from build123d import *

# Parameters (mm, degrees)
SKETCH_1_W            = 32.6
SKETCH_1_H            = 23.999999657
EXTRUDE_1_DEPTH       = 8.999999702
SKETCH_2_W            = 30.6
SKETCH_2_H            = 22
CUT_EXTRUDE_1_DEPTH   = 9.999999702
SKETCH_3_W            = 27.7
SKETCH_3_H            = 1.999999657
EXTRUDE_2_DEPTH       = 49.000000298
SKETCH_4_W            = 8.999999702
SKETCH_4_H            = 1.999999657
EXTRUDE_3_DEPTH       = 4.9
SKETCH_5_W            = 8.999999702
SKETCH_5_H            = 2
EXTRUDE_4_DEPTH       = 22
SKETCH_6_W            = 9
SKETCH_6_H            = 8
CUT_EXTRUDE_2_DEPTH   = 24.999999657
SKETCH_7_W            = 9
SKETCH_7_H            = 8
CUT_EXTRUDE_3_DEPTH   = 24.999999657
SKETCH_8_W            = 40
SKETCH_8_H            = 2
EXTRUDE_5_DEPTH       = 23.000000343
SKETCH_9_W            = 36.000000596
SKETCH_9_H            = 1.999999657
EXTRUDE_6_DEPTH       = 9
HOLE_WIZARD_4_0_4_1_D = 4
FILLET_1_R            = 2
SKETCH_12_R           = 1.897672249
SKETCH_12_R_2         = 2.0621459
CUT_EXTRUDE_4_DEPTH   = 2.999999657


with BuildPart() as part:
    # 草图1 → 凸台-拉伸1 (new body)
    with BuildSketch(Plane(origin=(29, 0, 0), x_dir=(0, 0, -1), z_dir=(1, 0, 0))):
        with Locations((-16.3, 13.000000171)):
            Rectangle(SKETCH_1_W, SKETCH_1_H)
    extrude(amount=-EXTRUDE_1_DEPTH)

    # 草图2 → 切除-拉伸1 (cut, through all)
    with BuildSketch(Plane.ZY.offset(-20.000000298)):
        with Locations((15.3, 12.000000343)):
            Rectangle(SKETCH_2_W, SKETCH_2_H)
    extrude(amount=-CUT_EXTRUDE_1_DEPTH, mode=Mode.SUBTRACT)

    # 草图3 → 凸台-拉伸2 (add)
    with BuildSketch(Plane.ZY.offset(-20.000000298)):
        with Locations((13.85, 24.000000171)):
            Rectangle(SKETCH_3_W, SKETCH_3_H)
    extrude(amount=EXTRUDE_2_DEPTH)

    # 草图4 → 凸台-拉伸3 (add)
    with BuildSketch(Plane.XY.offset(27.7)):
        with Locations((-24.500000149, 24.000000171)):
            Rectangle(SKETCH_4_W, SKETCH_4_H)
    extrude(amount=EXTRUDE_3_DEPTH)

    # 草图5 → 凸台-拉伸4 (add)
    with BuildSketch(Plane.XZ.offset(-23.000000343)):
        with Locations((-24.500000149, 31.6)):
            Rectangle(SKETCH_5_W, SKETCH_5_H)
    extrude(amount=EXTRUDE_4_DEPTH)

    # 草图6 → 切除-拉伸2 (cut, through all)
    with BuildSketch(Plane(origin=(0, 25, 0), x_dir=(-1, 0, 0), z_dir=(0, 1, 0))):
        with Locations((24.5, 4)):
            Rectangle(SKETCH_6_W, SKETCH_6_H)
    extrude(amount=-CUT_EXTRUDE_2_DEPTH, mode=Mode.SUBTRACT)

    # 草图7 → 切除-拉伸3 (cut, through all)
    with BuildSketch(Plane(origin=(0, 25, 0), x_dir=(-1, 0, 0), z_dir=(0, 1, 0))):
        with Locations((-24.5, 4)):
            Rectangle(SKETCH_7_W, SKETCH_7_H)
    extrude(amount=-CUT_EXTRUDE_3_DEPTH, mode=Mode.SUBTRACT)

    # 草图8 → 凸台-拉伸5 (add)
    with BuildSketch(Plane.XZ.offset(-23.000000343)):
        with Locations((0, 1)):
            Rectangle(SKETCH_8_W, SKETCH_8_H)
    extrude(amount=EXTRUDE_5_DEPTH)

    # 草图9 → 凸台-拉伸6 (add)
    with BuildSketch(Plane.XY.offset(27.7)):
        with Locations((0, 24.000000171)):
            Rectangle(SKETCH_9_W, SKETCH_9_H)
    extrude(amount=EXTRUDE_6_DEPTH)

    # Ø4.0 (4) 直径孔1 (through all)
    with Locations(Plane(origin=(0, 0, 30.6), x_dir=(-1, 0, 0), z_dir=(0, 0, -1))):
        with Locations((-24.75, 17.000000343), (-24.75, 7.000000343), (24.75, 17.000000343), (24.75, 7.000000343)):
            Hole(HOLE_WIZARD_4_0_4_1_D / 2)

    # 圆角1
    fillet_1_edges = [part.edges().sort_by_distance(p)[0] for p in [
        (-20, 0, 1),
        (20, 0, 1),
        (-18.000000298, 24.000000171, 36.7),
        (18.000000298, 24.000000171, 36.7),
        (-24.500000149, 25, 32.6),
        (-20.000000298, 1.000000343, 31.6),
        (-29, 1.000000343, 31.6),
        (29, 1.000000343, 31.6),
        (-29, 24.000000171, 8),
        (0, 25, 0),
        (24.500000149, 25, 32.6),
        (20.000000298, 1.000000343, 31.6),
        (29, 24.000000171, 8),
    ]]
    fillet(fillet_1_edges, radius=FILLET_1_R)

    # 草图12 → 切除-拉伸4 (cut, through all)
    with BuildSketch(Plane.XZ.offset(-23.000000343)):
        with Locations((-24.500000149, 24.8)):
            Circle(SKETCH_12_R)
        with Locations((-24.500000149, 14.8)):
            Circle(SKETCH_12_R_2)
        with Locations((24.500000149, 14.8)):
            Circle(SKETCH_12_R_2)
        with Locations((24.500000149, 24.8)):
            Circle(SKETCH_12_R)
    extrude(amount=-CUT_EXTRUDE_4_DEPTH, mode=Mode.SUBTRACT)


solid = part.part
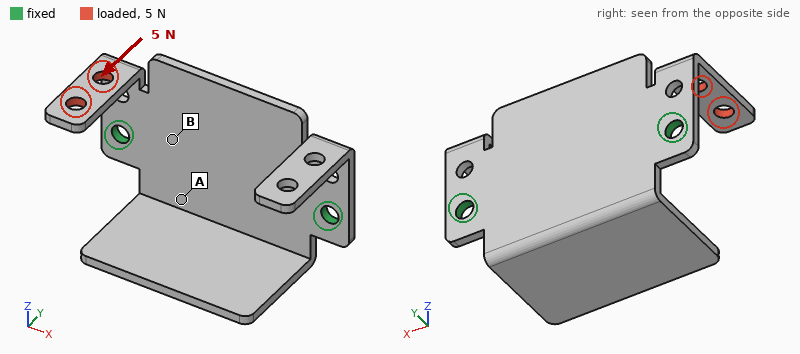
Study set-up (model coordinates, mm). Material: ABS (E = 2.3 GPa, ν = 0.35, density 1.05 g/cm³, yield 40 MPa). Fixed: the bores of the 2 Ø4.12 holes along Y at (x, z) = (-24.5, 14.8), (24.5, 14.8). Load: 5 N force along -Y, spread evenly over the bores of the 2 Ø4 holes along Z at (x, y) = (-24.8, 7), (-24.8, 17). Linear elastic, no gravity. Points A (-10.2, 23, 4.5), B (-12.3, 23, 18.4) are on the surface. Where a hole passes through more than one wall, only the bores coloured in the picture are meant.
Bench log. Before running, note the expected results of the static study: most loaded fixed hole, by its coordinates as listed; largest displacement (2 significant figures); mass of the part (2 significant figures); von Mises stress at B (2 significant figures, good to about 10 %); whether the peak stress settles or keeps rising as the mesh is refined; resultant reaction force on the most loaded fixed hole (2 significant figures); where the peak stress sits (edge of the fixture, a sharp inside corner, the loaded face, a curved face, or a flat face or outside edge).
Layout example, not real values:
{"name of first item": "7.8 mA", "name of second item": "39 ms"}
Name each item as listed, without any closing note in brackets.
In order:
{"most loaded fixed hole, by its coordinates as listed": "(-24.5, 14.8)", "largest displacement": "0.78 mm", "mass of the part": "6.4 g", "von Mises stress at B": "1.4 MPa", "whether the peak stress settles or keeps rising as the mesh is refined": "keeps rising", "resultant reaction force on the most loaded fixed hole": "5.2 N", "where the peak stress sits": "edge of the fixture"}
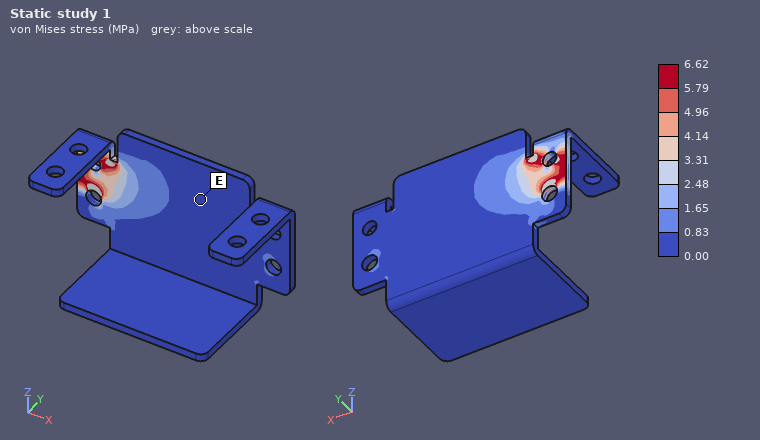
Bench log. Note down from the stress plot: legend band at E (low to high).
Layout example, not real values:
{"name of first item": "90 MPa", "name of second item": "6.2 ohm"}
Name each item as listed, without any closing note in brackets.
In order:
{"legend band at E": "0.00 to 0.83 MPa"}
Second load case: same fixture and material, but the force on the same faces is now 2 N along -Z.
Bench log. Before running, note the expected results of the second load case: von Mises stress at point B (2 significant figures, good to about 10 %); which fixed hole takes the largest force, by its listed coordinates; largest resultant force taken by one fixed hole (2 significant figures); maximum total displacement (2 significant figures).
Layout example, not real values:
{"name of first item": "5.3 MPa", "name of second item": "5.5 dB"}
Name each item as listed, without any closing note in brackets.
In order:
{"von Mises stress at point B": "0.59 MPa", "which fixed hole takes the largest force, by its listed coordinates": "(-24.5, 14.8)", "largest resultant force taken by one fixed hole": "2.0 N", "maximum total displacement": "0.77 mm"}
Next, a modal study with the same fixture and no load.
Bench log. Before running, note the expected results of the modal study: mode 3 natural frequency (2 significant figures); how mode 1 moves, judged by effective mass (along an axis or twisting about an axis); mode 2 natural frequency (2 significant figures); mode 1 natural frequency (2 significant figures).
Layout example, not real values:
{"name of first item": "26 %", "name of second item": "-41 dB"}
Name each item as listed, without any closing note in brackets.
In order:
{"mode 3 natural frequency": "500 Hz", "how mode 1 moves, judged by effective mass": "along Z", "mode 2 natural frequency": "490 Hz", "mode 1 natural frequency": "370 Hz"}
